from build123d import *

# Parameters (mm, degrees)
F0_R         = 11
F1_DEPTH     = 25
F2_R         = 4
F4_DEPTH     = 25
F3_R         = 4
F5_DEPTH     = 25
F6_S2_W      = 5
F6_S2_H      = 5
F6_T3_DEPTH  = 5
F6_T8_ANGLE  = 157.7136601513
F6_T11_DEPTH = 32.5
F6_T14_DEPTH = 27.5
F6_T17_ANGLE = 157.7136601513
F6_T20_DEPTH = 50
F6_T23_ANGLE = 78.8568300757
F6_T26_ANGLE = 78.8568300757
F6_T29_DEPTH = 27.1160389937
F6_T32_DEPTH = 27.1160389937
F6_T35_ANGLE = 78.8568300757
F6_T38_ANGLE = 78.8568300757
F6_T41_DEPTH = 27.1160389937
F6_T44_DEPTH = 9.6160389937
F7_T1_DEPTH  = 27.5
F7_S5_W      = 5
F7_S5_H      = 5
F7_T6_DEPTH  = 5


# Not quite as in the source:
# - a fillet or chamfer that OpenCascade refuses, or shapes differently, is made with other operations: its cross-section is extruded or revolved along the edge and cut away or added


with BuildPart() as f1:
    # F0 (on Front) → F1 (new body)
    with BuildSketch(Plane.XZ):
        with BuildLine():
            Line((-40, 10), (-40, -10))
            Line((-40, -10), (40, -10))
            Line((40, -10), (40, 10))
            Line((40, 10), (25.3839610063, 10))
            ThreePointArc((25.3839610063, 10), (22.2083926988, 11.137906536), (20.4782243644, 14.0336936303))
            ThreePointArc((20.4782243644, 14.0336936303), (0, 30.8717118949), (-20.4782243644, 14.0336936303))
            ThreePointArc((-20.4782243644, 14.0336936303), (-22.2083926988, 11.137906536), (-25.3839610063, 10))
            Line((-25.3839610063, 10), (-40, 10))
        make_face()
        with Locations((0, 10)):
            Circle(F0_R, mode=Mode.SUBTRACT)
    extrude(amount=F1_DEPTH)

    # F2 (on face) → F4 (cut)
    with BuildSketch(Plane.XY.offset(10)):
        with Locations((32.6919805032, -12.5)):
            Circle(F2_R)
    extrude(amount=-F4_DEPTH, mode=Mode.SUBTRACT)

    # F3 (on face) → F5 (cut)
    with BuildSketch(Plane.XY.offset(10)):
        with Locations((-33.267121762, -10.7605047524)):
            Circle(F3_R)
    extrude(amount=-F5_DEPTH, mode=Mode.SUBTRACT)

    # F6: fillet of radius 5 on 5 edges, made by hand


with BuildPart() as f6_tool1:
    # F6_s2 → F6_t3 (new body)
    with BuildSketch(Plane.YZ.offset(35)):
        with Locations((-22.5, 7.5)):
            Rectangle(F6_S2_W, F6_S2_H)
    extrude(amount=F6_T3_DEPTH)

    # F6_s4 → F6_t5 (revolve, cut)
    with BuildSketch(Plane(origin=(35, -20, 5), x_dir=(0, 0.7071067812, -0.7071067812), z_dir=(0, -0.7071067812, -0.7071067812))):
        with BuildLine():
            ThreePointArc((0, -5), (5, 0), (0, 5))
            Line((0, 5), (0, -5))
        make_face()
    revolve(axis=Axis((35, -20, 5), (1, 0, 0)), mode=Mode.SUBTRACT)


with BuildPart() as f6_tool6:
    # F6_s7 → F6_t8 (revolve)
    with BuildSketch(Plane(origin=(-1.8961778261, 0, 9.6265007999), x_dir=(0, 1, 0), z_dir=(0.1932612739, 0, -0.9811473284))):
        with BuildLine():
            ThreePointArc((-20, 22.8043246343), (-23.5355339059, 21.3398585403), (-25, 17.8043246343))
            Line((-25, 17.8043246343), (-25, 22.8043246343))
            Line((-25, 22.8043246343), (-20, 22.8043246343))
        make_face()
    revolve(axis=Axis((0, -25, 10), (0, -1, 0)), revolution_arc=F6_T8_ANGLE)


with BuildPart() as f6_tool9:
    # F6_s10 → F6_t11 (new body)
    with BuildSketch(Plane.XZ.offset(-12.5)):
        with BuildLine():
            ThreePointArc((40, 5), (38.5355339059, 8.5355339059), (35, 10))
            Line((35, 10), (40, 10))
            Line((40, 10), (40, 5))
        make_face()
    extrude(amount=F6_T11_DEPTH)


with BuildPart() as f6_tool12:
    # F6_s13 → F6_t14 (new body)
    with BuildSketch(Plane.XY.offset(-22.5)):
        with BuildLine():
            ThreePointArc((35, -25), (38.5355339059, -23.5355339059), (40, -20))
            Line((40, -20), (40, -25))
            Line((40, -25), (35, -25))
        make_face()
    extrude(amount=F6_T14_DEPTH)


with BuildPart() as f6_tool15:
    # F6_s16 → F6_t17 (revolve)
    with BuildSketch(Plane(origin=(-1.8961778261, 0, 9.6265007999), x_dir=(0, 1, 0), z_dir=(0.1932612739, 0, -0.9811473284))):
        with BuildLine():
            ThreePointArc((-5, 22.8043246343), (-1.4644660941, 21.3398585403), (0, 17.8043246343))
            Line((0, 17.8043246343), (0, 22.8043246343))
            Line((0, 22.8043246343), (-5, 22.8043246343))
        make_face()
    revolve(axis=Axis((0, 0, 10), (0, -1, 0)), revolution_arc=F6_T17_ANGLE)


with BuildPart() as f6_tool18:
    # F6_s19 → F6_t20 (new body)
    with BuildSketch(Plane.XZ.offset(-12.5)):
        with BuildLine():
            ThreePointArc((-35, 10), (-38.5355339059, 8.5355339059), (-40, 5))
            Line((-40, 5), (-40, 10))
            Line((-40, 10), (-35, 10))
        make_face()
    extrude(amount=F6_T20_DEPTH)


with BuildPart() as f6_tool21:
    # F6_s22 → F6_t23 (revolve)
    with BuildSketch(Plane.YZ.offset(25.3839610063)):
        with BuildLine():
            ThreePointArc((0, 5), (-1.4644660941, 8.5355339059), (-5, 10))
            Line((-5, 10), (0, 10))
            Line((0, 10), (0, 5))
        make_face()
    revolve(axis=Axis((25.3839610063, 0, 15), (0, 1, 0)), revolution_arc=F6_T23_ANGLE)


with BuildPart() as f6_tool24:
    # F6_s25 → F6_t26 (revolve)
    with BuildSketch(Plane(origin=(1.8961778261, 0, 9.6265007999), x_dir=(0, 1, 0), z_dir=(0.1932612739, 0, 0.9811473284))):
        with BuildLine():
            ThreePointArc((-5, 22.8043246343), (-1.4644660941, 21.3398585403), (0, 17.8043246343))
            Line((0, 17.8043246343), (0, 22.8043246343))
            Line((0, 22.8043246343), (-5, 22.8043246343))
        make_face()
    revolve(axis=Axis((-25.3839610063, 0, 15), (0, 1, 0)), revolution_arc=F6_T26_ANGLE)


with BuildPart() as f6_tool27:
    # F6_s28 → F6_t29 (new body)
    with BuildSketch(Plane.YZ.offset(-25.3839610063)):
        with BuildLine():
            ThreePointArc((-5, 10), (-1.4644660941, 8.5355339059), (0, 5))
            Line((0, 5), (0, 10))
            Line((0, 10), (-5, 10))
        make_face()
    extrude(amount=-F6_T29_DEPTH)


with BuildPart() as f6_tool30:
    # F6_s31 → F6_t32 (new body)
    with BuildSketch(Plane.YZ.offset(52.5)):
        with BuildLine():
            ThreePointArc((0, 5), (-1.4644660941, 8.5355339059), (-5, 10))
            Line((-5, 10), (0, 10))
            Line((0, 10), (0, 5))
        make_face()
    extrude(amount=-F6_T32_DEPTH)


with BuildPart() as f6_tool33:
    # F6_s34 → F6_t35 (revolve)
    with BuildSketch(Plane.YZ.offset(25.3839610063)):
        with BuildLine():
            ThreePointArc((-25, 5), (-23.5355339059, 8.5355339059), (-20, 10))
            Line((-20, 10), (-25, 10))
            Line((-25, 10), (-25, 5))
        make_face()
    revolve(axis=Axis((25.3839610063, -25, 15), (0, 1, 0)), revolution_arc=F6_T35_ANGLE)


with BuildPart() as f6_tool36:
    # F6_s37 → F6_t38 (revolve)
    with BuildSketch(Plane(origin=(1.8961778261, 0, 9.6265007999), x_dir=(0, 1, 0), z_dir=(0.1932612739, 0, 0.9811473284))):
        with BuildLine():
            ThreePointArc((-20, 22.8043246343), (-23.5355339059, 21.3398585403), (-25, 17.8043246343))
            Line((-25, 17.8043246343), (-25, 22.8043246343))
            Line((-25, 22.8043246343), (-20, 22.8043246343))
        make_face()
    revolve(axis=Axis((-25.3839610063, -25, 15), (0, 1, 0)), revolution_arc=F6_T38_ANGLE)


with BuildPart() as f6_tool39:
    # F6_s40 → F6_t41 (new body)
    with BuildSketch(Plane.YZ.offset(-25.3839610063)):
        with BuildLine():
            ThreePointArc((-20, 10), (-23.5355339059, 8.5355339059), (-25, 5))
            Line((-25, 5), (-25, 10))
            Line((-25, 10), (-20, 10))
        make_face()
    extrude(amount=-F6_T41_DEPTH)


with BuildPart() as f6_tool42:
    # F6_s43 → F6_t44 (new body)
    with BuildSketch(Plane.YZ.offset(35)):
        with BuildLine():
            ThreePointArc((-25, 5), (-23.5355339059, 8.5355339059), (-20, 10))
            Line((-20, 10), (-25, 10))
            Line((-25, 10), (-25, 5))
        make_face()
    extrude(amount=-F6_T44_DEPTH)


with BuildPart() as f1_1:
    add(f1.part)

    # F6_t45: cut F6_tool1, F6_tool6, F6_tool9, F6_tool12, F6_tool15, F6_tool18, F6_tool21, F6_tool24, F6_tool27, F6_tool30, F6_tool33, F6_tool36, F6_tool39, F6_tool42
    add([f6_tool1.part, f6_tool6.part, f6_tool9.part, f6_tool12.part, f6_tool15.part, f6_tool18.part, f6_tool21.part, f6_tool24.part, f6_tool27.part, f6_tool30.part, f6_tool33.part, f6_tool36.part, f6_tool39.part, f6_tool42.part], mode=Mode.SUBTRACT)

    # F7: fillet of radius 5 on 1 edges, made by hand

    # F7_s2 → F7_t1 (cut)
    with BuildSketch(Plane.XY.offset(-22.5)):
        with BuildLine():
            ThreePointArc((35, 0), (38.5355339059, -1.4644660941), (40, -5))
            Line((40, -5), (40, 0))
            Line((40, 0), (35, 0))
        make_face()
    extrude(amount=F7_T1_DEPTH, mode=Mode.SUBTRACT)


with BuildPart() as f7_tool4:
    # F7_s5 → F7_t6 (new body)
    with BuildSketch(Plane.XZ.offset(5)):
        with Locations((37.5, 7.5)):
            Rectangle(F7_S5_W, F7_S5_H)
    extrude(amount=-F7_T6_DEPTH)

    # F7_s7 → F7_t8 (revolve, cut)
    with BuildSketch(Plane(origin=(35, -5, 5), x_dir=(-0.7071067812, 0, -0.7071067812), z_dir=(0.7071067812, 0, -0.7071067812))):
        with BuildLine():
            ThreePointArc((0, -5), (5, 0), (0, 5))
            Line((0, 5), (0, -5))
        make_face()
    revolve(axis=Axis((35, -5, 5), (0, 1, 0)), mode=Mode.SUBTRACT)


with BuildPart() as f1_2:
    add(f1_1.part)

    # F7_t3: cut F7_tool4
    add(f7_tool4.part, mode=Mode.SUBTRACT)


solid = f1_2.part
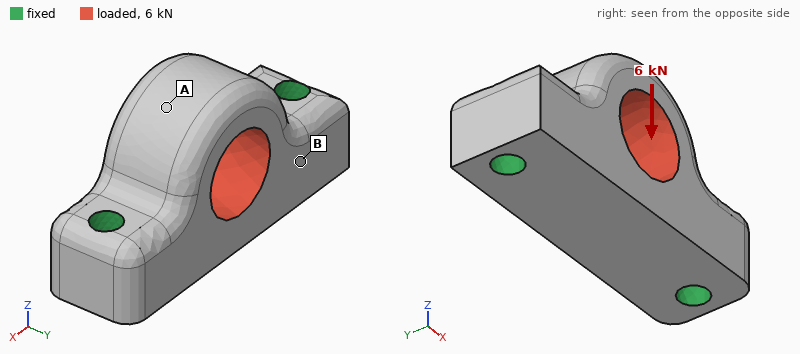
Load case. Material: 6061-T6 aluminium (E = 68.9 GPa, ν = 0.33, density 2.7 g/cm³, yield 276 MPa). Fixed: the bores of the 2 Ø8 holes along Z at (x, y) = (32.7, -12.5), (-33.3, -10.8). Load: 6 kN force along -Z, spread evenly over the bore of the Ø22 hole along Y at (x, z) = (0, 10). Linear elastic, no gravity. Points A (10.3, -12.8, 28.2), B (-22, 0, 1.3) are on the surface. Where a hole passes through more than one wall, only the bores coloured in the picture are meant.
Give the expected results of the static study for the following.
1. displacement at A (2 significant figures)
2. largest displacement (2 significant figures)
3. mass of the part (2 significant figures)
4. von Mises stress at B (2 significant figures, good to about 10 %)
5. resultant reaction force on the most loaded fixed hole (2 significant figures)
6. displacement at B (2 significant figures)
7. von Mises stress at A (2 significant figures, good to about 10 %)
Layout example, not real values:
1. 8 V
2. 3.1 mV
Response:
1. 7.3 µm
2. 11 µm
3. 120 g
4. 12 MPa
5. 3.0 kN
6. 3.7 µm
7. 3.9 MPa
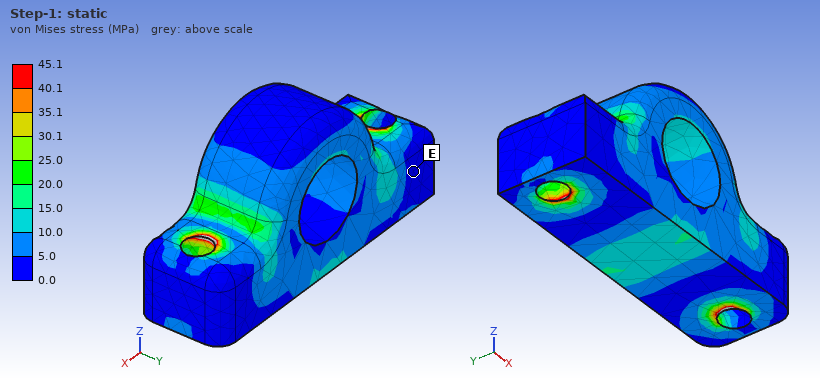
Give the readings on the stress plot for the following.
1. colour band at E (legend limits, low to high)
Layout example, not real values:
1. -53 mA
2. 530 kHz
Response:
1. 0.0 to 5.0 MPa
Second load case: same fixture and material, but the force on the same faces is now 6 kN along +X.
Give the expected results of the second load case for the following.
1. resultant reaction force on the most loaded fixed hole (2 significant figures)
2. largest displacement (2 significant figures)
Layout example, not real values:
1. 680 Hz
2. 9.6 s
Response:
1. 3.1 kN
2. 8.0 µm
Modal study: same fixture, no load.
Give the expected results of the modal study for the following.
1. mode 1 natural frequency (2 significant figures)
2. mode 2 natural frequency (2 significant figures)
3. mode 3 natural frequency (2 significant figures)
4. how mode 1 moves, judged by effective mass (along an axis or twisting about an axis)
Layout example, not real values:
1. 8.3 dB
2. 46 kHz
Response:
1. 9700 Hz
2. 16 kHz
3. 17 kHz
4. along Y
